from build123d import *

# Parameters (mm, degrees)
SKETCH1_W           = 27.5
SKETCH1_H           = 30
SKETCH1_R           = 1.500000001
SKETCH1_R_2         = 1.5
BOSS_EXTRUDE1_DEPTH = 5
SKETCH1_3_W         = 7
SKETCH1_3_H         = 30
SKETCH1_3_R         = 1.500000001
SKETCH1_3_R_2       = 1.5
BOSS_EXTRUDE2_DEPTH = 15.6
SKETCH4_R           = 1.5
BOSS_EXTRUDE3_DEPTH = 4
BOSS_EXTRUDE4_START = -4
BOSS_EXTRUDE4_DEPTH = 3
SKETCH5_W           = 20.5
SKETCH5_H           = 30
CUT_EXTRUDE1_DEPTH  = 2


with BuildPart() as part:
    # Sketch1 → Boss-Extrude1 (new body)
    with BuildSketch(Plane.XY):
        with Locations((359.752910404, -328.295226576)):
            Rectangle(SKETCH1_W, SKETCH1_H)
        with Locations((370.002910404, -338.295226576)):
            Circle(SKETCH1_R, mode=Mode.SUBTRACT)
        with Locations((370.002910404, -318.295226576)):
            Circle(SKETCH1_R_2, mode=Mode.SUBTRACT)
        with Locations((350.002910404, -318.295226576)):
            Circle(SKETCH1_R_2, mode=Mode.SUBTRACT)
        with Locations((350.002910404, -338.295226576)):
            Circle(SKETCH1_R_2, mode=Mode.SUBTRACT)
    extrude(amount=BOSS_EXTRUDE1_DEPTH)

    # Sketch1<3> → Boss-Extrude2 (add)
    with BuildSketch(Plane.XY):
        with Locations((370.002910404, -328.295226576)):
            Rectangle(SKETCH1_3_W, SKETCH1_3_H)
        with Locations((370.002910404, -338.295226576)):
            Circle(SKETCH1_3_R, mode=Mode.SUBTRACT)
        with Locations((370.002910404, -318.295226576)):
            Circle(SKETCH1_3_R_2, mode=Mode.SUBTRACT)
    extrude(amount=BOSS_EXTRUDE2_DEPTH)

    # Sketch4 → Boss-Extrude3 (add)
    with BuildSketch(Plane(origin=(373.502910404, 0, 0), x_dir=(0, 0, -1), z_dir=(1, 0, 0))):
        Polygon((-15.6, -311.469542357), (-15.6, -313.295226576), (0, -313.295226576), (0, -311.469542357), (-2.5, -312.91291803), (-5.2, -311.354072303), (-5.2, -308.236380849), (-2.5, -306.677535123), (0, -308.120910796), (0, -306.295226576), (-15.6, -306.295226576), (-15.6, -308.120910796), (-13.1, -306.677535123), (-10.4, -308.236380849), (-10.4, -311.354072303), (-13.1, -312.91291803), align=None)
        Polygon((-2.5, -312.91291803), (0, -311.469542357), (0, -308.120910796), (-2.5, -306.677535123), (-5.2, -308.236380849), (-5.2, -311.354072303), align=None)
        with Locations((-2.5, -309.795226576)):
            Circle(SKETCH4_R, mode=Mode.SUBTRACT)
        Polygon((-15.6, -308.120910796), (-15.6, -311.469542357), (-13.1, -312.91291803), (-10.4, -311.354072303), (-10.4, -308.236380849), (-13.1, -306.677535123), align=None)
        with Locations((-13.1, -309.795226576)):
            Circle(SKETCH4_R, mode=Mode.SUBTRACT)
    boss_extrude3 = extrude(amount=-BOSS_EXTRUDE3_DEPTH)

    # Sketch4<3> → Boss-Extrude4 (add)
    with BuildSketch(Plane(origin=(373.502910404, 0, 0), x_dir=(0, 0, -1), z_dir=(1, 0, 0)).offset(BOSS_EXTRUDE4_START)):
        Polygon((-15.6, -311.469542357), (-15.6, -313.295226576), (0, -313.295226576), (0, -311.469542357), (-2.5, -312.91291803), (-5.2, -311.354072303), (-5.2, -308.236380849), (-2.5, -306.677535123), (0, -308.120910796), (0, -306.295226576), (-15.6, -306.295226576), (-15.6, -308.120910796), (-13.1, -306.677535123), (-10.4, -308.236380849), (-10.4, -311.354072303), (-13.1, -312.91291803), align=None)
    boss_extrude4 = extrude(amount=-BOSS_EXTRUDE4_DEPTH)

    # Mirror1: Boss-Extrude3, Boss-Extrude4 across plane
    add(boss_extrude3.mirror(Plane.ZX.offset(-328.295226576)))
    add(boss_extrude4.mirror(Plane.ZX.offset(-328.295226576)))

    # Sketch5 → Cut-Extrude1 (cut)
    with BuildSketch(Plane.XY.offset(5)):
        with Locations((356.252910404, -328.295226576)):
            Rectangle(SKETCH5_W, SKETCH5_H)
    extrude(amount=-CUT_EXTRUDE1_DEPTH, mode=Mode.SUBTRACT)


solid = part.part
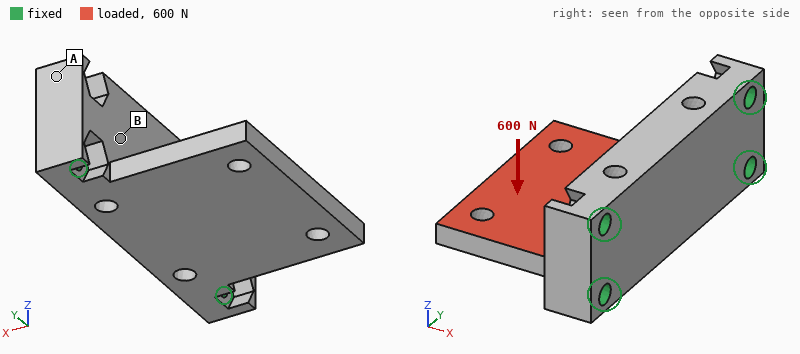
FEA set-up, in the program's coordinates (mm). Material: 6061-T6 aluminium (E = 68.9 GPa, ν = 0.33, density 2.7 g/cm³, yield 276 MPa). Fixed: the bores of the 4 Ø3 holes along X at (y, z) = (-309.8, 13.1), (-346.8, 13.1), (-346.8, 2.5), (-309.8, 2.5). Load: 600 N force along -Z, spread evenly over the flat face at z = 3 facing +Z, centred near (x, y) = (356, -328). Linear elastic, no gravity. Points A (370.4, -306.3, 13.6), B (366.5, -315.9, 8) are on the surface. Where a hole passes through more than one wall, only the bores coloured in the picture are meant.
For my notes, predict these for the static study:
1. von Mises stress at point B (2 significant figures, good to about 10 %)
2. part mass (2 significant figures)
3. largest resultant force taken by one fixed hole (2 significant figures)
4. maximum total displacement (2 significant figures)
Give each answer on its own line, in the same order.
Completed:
26 MPa
16 g
510 N
0.21 mm
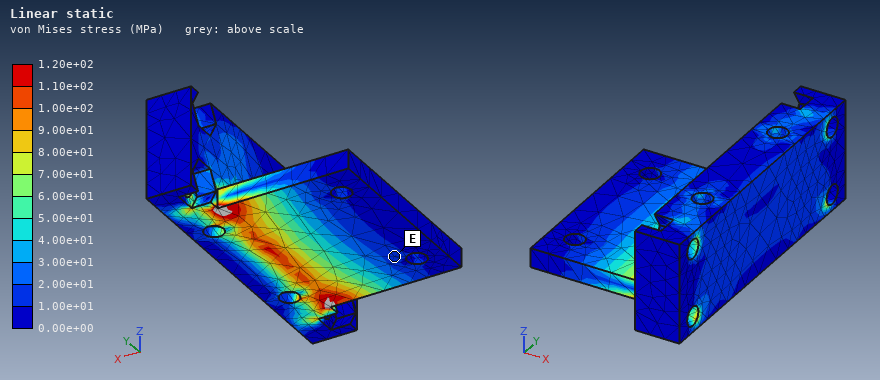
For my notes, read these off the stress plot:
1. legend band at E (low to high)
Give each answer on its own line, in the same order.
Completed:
1.00e+01 to 2.00e+01 MPa
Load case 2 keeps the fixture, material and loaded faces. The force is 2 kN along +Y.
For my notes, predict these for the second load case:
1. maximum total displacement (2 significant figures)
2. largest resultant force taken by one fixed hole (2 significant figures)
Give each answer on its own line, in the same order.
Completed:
69 µm
1.1 kN
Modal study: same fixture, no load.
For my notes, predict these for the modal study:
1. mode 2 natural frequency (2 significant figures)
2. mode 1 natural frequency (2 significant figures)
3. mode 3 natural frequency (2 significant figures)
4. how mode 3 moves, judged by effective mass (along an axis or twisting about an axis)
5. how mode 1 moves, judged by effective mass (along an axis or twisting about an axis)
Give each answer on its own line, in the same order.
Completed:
9500 Hz
4800 Hz
19 kHz
along X
along Z
